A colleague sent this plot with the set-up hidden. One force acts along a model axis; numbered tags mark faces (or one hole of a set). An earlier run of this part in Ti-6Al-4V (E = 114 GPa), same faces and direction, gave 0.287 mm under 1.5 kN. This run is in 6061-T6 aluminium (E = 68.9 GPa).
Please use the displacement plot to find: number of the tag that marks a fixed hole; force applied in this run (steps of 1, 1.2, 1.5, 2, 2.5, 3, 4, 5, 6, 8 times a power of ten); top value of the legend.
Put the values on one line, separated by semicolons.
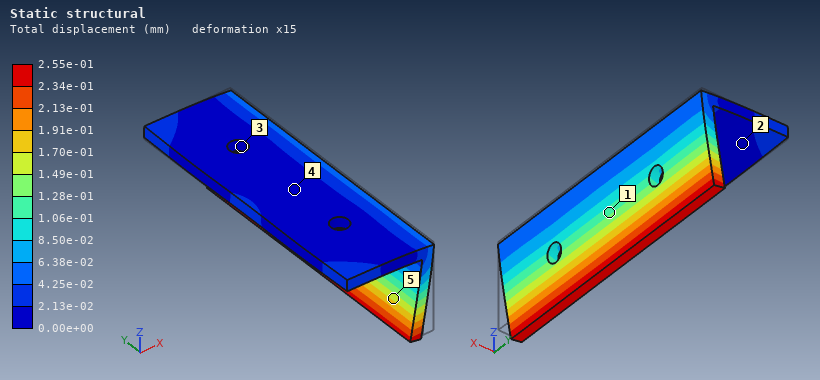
3; 800 N; 2.55e-01 mm
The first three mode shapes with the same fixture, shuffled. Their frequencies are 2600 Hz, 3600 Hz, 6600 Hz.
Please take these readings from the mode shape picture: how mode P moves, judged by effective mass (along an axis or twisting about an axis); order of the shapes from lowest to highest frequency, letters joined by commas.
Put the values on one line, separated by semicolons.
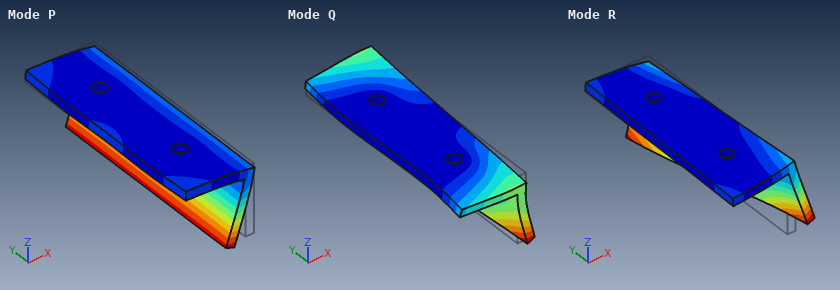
along X; P, R, Q
